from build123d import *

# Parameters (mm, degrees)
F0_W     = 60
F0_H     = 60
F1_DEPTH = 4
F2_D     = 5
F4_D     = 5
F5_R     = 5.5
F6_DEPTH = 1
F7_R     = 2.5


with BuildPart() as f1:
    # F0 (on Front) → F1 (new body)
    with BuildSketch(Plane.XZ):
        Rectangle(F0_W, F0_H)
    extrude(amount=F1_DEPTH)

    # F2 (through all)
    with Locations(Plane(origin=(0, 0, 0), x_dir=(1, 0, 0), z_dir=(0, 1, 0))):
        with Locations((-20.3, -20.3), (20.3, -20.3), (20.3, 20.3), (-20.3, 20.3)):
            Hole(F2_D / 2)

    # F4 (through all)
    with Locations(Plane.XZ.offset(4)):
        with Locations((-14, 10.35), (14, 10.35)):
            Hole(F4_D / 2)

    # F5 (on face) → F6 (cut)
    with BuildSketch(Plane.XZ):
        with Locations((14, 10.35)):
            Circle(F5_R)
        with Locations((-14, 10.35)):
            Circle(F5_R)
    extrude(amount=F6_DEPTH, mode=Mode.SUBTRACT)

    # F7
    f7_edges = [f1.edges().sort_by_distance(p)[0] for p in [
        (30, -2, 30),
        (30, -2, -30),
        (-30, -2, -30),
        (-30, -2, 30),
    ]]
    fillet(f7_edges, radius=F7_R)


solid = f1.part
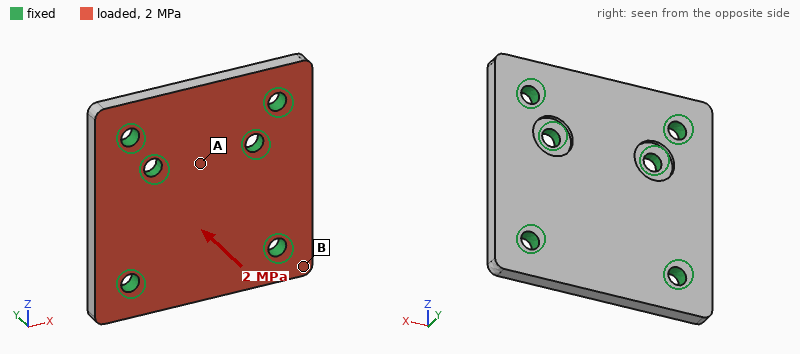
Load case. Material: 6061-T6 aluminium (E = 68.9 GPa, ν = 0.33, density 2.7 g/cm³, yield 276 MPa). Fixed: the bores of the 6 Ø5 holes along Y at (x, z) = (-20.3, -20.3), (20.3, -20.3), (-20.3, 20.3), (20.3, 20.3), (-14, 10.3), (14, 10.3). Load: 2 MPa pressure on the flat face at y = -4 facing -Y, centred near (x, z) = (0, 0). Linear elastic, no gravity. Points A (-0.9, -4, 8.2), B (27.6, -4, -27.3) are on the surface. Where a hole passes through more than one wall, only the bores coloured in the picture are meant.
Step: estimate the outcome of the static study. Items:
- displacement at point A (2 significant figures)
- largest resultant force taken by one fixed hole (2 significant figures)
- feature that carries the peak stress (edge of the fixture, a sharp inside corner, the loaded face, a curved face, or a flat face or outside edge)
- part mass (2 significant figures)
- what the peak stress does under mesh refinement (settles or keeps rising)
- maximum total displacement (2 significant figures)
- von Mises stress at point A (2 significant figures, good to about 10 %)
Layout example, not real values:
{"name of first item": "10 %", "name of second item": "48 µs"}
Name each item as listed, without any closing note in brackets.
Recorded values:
{"displacement at point A": "17 µm", "largest resultant force taken by one fixed hole": "1.5 kN", "feature that carries the peak stress": "edge of the fixture", "part mass": "37 g", "what the peak stress does under mesh refinement": "keeps rising", "maximum total displacement": "41 µm", "von Mises stress at point A": "37 MPa"}
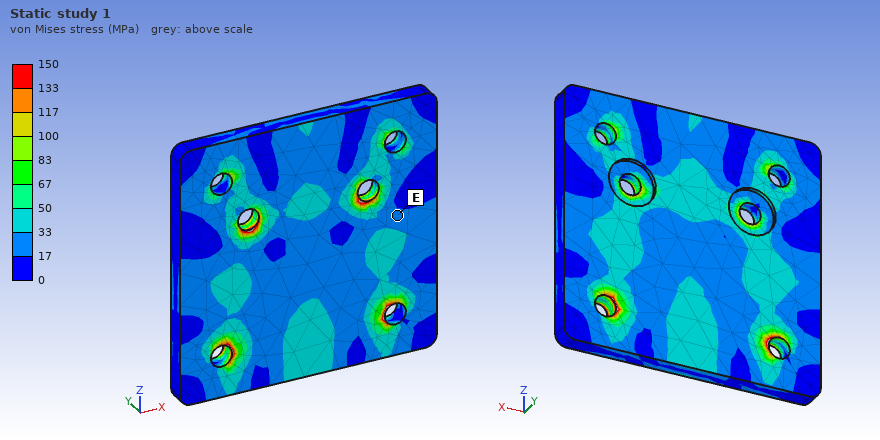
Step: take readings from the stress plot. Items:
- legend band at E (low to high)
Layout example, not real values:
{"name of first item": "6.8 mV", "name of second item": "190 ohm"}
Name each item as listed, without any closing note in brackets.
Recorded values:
{"legend band at E": "17 to 33 MPa"}
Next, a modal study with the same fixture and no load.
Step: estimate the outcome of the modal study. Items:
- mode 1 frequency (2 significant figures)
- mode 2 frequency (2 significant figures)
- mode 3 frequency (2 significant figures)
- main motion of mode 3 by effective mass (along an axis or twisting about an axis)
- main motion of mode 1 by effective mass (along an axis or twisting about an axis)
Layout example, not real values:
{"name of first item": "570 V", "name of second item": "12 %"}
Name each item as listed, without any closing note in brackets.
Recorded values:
{"mode 1 frequency": "13 kHz", "mode 2 frequency": "14 kHz", "mode 3 frequency": "16 kHz", "main motion of mode 3 by effective mass": "along Y", "main motion of mode 1 by effective mass": "along Y"}
